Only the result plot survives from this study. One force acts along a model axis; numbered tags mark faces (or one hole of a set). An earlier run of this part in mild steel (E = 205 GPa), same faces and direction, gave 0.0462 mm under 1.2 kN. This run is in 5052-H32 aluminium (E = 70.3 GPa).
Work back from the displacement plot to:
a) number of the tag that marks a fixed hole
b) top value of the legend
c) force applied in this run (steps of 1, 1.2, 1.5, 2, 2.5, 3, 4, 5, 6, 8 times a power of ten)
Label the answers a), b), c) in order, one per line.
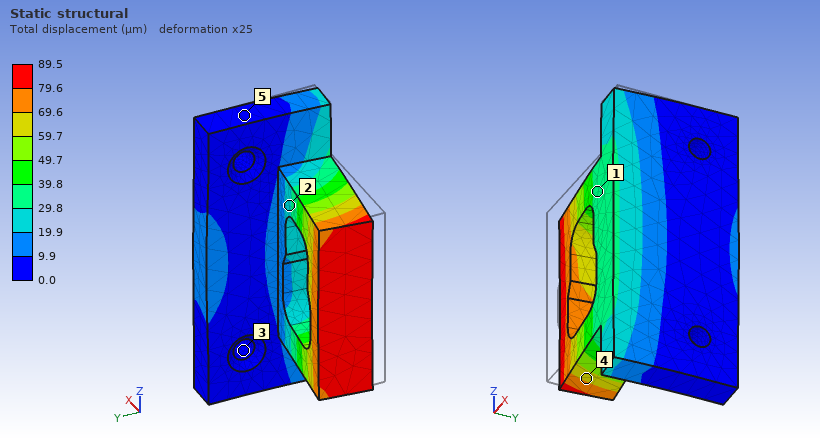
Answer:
a) 3
b) 89.5 µm
c) 800 N
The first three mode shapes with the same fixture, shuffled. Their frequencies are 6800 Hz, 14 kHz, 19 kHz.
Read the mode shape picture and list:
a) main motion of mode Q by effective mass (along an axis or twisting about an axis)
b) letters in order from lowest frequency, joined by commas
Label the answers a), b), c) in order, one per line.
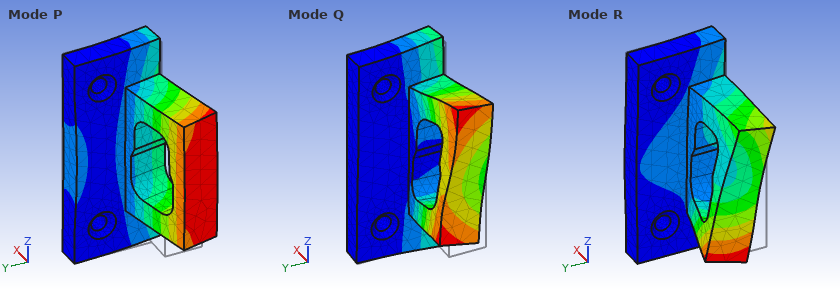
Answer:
a) along Z
b) P, Q, R
